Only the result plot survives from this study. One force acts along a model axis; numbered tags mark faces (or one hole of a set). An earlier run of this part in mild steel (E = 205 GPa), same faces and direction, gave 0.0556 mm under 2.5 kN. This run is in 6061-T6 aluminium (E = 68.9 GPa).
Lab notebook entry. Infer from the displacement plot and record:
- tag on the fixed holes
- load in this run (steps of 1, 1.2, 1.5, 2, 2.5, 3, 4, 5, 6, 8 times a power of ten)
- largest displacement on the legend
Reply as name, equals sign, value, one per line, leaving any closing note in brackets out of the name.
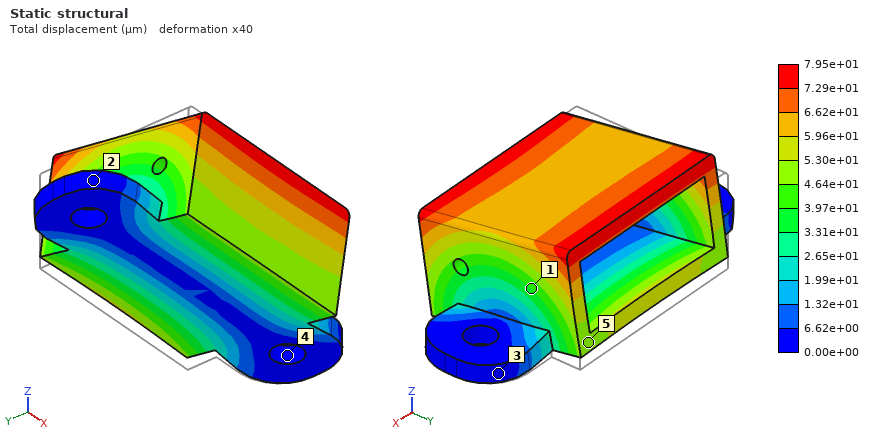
tag on the fixed holes = 4
load in this run = 1.2 kN
largest displacement on the legend = 7.95e+01 µm
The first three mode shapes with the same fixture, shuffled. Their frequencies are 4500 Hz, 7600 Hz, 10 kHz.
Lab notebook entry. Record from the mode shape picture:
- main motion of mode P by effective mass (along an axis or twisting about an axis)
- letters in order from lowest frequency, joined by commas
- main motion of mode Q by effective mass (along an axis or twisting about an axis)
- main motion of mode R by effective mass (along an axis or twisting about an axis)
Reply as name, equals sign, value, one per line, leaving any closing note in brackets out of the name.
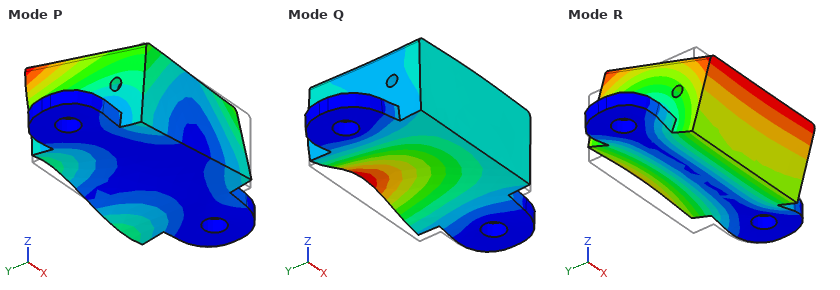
main motion of mode P by effective mass = along X
letters in order from lowest frequency, joined by commas = R, P, Q
main motion of mode Q by effective mass = along Z
main motion of mode R by effective mass = along Y
